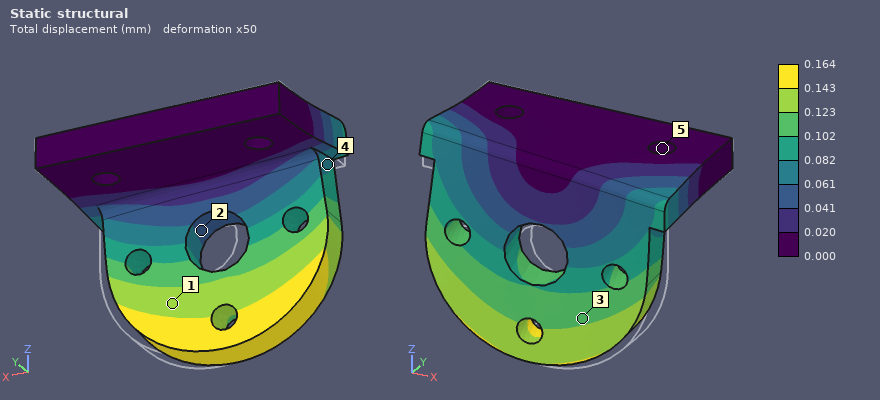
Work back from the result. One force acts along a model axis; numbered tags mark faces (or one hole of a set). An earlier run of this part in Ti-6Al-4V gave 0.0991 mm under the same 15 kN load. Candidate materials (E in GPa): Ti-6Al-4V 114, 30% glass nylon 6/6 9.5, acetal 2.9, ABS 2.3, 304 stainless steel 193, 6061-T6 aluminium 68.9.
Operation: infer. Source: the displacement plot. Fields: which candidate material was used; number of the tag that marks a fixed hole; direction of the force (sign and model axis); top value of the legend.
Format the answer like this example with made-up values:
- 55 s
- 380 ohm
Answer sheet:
- 6061-T6 aluminium
- 5
- -X
- 0.164 mm
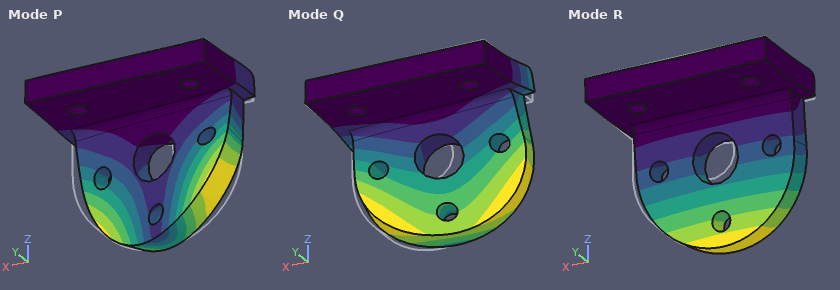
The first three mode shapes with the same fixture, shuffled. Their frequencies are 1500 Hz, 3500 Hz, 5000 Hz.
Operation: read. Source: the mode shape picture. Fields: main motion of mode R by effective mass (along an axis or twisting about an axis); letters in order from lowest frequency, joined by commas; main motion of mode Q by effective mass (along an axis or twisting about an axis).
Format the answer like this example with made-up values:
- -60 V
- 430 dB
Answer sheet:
- along Y
- R, Q, P
- along X
